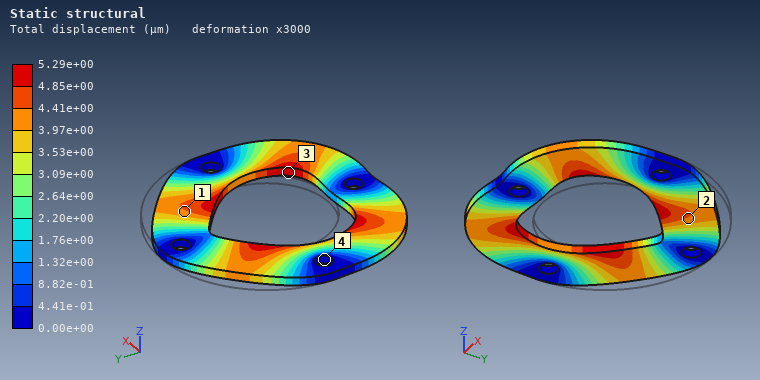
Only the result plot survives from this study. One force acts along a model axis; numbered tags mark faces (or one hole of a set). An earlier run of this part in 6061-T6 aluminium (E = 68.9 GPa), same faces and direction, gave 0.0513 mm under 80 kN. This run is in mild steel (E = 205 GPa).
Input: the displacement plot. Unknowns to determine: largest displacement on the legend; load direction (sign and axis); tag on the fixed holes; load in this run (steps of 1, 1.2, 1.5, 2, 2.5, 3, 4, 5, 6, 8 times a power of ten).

5.29e+00 µm
-Y
4
25 kN
